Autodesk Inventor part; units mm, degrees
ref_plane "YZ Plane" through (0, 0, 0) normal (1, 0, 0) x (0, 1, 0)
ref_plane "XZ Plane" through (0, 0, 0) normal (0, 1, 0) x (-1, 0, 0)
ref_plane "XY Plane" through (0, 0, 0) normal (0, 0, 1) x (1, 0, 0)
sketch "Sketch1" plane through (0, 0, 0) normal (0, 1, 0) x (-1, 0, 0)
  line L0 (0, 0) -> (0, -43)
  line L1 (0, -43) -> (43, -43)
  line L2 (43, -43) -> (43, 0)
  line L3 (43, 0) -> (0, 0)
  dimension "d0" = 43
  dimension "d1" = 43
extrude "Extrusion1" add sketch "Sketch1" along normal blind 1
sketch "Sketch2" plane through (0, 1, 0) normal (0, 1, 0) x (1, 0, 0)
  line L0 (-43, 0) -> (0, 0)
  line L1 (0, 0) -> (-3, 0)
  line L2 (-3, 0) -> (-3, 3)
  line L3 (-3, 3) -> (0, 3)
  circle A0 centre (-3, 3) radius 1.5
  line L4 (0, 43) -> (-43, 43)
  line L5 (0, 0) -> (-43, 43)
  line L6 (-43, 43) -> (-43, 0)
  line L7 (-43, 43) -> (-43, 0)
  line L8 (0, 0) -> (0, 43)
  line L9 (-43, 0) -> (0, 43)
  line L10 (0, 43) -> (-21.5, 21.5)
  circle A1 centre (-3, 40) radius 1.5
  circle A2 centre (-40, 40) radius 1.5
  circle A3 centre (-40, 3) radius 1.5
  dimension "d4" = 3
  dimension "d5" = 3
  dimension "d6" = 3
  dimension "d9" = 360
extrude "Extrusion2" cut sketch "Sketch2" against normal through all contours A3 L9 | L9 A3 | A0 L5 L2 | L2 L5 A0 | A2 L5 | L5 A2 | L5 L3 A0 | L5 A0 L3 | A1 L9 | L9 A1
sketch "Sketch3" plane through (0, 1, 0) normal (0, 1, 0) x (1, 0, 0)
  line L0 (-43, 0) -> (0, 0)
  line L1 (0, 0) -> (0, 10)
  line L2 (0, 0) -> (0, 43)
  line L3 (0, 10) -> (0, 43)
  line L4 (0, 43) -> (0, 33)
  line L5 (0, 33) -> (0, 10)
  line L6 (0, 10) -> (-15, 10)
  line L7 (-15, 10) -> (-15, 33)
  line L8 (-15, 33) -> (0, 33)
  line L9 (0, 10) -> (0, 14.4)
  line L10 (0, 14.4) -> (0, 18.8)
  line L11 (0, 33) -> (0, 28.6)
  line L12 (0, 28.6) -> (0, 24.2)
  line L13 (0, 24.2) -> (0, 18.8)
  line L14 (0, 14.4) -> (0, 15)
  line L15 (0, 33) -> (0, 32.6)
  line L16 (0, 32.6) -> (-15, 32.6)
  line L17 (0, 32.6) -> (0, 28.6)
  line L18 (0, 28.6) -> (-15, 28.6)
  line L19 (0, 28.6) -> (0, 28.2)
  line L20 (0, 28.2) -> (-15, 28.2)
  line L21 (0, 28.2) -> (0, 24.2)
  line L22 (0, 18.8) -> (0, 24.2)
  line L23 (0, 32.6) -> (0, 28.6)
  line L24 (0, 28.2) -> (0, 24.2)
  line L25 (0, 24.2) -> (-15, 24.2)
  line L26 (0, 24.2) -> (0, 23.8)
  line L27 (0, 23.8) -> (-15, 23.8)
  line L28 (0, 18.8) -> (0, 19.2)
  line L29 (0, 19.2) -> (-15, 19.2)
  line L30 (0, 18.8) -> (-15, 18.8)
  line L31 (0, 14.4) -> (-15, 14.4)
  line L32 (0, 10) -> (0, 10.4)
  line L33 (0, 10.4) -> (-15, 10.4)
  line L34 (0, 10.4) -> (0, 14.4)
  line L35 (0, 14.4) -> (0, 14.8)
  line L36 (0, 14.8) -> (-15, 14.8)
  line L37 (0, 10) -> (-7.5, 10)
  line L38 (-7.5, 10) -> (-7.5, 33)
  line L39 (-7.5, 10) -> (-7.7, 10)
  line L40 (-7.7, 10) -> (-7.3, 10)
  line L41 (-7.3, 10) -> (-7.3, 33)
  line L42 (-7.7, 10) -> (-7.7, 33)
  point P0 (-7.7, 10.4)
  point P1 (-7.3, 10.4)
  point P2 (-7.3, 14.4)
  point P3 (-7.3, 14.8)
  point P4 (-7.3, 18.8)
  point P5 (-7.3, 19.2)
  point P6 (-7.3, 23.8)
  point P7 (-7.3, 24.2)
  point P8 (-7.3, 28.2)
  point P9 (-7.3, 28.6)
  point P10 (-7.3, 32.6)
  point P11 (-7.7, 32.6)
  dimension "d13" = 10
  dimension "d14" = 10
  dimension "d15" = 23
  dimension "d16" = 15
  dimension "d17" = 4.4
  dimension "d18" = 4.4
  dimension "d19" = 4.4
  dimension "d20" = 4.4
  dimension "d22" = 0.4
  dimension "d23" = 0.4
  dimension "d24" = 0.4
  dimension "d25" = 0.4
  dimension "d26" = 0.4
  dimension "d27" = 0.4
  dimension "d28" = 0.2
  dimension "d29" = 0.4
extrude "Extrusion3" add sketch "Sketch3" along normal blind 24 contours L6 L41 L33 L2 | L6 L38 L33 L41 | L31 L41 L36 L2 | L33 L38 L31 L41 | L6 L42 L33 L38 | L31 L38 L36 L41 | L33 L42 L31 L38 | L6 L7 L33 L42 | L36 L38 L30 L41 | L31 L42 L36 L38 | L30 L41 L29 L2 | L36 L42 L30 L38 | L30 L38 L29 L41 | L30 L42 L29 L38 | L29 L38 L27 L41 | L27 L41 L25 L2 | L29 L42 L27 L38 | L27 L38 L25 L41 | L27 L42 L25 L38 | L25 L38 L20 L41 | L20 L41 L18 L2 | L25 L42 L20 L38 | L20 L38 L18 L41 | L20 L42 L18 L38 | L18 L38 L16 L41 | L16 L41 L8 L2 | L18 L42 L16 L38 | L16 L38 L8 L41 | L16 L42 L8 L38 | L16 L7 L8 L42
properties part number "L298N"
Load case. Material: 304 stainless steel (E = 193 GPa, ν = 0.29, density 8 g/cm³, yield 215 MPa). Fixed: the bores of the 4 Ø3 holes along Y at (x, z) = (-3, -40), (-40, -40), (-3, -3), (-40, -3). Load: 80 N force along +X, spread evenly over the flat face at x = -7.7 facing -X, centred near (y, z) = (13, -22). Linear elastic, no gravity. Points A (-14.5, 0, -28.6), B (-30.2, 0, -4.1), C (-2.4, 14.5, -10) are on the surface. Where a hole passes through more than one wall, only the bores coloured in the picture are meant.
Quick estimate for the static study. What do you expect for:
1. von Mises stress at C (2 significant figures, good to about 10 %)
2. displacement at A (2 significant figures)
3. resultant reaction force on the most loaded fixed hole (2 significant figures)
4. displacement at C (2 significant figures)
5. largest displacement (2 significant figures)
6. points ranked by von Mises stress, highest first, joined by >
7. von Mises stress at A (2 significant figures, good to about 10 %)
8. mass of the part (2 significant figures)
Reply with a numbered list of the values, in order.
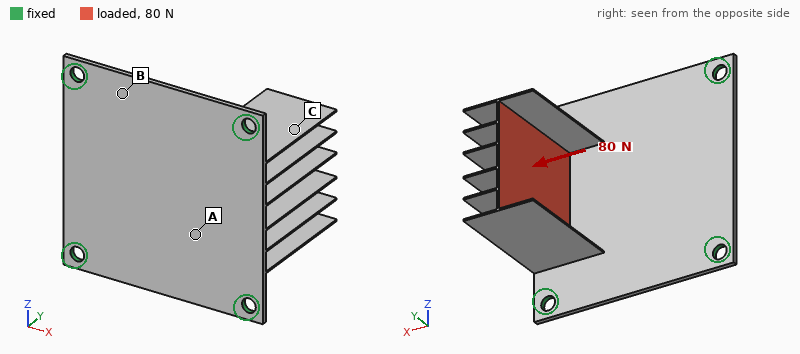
1. 26 MPa
2. 0.032 mm
3. 29 N
4. 0.060 mm
5. 0.18 mm
6. A > C > B
7. 47 MPa
8. 21 g
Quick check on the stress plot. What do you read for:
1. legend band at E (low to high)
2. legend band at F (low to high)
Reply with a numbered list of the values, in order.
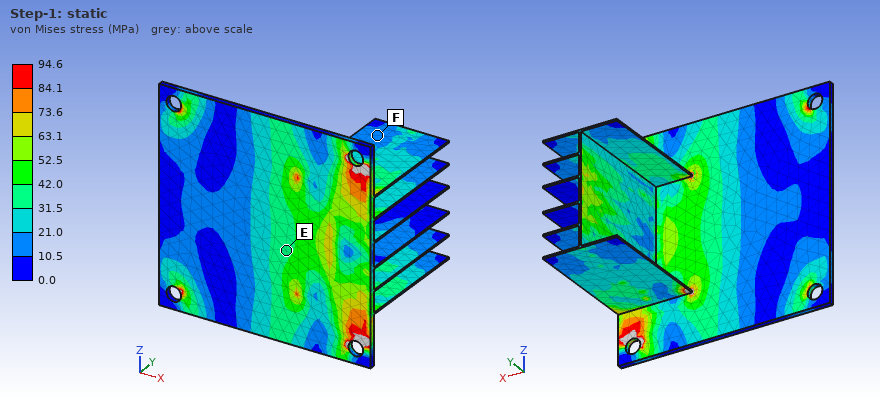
1. 31.5 to 42.0 MPa
2. 10.5 to 21.0 MPa
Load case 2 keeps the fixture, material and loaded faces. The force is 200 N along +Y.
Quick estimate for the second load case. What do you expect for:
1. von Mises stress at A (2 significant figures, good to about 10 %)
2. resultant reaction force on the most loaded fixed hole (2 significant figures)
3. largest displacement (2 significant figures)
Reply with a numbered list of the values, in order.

1. 32 MPa
2. 93 N
3. 55 µm
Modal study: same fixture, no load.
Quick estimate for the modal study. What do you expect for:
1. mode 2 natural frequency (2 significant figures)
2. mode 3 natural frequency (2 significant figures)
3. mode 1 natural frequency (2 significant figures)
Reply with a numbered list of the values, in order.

1. 2900 Hz
2. 2900 Hz
3. 1700 Hz
